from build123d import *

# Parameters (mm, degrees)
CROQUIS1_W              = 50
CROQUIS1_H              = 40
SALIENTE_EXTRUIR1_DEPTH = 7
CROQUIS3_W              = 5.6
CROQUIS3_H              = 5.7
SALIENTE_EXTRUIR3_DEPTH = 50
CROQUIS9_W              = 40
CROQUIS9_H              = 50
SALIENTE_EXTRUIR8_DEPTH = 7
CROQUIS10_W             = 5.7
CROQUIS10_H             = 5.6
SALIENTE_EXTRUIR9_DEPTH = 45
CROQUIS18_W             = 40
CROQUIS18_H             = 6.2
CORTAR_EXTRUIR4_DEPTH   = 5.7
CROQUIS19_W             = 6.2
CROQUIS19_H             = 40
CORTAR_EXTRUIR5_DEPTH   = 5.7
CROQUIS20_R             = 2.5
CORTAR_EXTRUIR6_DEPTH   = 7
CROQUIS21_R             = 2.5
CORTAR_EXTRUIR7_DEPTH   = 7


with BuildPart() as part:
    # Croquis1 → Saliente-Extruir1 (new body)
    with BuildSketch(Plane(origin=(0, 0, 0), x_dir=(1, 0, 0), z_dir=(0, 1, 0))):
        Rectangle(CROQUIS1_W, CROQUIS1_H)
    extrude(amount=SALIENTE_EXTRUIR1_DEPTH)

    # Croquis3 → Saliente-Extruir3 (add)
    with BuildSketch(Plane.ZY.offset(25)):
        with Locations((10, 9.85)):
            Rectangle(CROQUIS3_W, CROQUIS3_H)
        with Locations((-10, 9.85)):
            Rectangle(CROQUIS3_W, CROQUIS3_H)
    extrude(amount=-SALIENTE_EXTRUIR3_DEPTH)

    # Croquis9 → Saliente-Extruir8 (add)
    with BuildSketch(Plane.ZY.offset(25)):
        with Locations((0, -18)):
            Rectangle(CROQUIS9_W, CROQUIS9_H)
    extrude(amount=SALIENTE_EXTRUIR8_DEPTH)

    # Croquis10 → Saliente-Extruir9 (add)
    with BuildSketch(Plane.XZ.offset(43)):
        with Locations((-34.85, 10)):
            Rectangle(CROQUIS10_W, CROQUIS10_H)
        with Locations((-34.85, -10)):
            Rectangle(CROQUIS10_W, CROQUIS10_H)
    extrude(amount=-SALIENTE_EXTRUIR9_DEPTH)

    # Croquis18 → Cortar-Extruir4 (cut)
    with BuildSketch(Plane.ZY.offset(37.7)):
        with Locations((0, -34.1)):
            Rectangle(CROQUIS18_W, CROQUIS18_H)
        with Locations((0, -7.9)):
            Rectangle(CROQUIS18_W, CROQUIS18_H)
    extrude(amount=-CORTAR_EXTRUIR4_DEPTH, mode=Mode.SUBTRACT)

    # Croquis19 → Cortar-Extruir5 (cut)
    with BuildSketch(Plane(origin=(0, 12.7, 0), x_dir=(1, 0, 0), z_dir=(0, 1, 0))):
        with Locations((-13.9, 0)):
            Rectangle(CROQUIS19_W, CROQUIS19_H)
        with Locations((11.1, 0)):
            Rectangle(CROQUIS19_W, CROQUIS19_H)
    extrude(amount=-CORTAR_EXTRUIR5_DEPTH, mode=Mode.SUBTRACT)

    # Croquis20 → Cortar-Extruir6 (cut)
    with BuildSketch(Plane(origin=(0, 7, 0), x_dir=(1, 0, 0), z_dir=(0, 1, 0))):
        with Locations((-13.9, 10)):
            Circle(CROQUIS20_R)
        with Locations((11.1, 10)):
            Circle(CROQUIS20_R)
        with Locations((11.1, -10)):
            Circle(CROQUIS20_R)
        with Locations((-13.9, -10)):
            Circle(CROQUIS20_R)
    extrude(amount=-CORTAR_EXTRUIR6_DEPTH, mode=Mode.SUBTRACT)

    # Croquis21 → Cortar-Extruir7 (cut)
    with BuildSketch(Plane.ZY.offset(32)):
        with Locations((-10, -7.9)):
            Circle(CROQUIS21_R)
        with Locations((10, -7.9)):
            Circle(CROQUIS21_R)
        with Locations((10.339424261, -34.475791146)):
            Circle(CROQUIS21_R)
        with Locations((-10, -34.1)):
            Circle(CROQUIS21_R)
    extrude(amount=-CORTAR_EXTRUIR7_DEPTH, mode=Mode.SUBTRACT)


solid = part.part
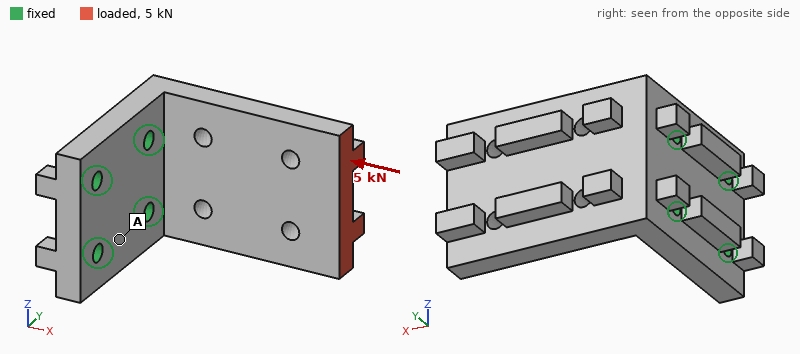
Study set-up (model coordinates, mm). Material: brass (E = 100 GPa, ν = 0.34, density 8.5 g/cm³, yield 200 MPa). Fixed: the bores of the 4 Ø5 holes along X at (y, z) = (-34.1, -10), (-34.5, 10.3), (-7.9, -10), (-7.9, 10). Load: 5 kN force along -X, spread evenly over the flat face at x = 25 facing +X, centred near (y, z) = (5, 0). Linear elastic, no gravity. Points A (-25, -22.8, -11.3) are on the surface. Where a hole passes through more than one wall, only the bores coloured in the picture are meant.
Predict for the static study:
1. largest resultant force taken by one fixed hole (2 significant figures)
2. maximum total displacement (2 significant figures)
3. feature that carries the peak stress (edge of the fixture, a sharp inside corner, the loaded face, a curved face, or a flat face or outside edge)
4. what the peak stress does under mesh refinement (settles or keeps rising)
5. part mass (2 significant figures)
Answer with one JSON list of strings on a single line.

["2.7 kN", "0.25 mm", "edge of the fixture", "keeps rising", "270 g"]
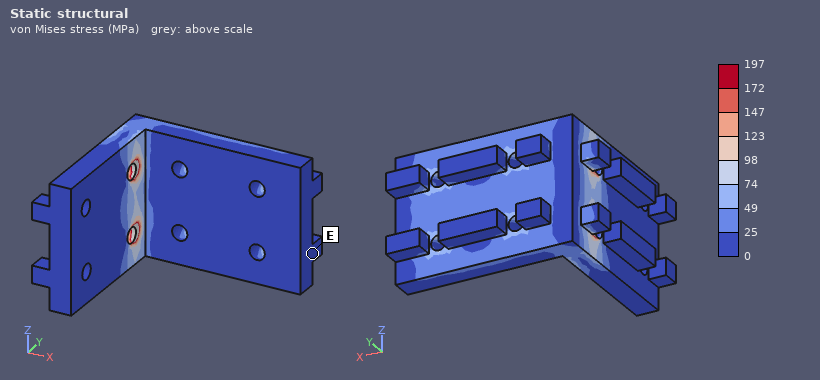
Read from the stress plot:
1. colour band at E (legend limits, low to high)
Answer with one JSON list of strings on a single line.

["0 to 25 MPa"]
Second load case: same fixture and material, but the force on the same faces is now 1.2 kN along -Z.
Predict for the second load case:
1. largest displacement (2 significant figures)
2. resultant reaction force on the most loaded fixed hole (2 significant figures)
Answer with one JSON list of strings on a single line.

["100 µm", "2.6 kN"]
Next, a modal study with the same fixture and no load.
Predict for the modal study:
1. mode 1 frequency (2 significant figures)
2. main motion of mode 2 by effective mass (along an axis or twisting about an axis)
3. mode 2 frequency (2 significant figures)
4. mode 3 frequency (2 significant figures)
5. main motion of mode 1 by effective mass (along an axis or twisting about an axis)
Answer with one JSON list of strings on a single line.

["1000 Hz", "along Z", "2500 Hz", "3600 Hz", "along Y"]
